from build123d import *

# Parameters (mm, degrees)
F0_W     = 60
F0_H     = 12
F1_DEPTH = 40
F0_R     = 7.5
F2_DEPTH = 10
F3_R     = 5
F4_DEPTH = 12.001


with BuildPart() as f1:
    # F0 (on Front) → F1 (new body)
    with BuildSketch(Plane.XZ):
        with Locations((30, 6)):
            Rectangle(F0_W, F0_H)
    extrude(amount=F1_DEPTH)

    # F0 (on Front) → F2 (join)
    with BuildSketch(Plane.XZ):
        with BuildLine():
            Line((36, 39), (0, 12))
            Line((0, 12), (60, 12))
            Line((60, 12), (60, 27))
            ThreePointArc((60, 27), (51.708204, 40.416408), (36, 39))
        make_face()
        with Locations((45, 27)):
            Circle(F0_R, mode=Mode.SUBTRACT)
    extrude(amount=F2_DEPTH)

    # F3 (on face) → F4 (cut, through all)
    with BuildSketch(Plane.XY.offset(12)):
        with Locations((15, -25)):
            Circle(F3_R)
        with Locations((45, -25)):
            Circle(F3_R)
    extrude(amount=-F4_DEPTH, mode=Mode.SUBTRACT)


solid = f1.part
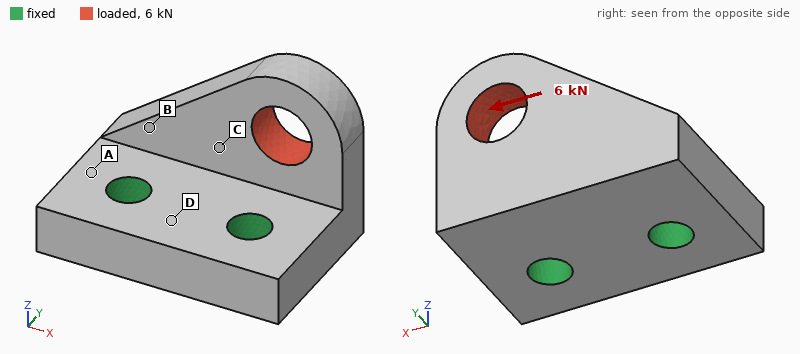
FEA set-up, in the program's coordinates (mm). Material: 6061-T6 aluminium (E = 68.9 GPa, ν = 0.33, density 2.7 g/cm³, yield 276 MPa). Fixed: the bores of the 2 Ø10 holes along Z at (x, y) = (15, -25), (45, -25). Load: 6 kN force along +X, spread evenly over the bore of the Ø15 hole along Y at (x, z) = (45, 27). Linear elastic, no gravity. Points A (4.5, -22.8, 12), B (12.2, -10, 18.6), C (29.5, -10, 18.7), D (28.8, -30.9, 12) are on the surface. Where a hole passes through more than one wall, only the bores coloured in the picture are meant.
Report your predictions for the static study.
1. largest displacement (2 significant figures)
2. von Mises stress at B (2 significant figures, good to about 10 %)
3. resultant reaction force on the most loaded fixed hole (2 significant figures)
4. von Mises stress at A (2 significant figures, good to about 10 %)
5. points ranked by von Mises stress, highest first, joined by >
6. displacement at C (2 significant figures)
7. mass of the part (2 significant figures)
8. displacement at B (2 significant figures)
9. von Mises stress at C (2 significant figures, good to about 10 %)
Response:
75 µm
45 MPa
5.1 kN
19 MPa
B > C > A > D
24 µm
99 g
28 µm
28 MPa
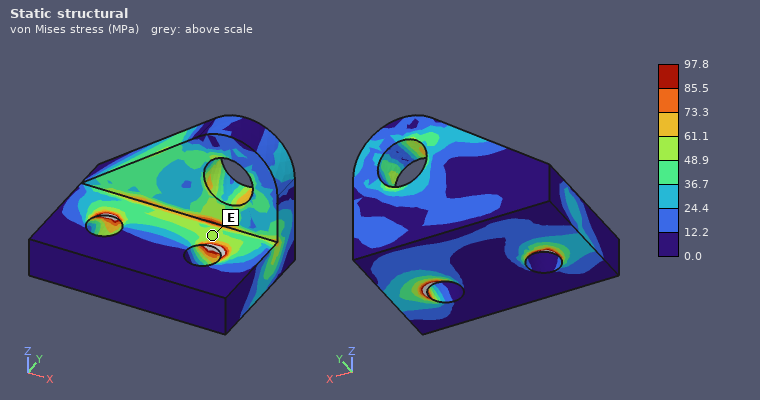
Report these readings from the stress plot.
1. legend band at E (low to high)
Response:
48.9 to 61.1 MPa
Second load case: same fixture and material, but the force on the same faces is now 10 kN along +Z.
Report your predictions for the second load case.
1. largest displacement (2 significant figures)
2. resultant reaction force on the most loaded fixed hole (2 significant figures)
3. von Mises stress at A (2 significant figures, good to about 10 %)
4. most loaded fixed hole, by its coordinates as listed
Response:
0.17 mm
8.6 kN
23 MPa
(45, -25)
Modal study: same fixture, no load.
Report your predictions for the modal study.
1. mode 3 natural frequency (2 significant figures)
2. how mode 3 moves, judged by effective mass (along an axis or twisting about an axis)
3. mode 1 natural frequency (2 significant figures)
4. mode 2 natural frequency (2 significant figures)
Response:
13 kHz
along Z
6100 Hz
10 kHz
